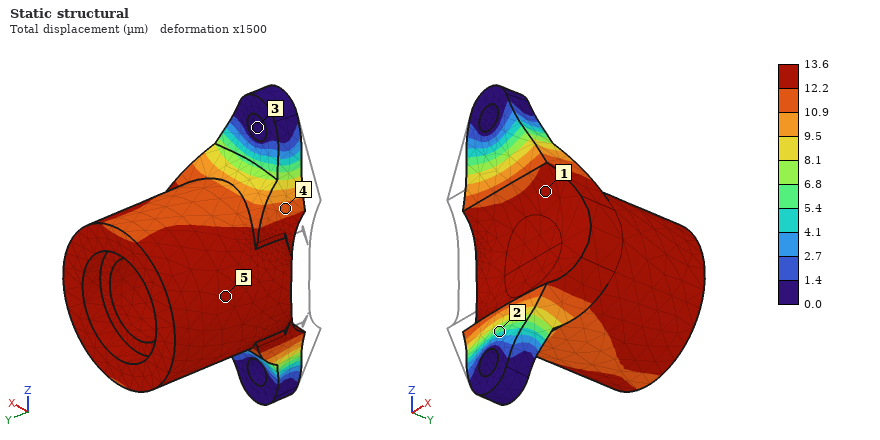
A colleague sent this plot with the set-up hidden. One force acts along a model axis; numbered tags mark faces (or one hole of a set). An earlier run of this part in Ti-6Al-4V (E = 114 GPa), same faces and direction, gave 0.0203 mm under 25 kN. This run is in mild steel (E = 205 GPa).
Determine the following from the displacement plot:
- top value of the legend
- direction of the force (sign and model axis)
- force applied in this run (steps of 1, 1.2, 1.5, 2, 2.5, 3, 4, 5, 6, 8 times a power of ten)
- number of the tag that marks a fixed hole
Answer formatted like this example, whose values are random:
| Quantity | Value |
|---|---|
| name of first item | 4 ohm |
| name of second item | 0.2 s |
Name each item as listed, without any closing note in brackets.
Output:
| Quantity | Value |
|---|---|
| top value of the legend | 13.6 µm |
| direction of the force | +Y |
| force applied in this run | 30 kN |
| number of the tag that marks a fixed hole | 3 |
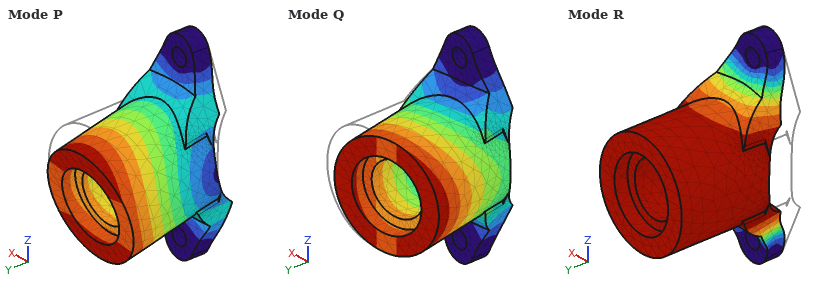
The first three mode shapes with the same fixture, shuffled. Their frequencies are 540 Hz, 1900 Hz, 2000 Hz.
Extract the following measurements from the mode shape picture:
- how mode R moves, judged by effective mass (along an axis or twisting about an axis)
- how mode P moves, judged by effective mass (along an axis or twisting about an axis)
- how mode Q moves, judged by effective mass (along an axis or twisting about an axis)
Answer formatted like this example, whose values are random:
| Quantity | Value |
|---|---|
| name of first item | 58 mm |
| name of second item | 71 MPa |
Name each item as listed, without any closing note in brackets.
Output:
| Quantity | Value |
|---|---|
| how mode R moves, judged by effective mass | along Y |
| how mode P moves, judged by effective mass | along Z |
| how mode Q moves, judged by effective mass | along X |
